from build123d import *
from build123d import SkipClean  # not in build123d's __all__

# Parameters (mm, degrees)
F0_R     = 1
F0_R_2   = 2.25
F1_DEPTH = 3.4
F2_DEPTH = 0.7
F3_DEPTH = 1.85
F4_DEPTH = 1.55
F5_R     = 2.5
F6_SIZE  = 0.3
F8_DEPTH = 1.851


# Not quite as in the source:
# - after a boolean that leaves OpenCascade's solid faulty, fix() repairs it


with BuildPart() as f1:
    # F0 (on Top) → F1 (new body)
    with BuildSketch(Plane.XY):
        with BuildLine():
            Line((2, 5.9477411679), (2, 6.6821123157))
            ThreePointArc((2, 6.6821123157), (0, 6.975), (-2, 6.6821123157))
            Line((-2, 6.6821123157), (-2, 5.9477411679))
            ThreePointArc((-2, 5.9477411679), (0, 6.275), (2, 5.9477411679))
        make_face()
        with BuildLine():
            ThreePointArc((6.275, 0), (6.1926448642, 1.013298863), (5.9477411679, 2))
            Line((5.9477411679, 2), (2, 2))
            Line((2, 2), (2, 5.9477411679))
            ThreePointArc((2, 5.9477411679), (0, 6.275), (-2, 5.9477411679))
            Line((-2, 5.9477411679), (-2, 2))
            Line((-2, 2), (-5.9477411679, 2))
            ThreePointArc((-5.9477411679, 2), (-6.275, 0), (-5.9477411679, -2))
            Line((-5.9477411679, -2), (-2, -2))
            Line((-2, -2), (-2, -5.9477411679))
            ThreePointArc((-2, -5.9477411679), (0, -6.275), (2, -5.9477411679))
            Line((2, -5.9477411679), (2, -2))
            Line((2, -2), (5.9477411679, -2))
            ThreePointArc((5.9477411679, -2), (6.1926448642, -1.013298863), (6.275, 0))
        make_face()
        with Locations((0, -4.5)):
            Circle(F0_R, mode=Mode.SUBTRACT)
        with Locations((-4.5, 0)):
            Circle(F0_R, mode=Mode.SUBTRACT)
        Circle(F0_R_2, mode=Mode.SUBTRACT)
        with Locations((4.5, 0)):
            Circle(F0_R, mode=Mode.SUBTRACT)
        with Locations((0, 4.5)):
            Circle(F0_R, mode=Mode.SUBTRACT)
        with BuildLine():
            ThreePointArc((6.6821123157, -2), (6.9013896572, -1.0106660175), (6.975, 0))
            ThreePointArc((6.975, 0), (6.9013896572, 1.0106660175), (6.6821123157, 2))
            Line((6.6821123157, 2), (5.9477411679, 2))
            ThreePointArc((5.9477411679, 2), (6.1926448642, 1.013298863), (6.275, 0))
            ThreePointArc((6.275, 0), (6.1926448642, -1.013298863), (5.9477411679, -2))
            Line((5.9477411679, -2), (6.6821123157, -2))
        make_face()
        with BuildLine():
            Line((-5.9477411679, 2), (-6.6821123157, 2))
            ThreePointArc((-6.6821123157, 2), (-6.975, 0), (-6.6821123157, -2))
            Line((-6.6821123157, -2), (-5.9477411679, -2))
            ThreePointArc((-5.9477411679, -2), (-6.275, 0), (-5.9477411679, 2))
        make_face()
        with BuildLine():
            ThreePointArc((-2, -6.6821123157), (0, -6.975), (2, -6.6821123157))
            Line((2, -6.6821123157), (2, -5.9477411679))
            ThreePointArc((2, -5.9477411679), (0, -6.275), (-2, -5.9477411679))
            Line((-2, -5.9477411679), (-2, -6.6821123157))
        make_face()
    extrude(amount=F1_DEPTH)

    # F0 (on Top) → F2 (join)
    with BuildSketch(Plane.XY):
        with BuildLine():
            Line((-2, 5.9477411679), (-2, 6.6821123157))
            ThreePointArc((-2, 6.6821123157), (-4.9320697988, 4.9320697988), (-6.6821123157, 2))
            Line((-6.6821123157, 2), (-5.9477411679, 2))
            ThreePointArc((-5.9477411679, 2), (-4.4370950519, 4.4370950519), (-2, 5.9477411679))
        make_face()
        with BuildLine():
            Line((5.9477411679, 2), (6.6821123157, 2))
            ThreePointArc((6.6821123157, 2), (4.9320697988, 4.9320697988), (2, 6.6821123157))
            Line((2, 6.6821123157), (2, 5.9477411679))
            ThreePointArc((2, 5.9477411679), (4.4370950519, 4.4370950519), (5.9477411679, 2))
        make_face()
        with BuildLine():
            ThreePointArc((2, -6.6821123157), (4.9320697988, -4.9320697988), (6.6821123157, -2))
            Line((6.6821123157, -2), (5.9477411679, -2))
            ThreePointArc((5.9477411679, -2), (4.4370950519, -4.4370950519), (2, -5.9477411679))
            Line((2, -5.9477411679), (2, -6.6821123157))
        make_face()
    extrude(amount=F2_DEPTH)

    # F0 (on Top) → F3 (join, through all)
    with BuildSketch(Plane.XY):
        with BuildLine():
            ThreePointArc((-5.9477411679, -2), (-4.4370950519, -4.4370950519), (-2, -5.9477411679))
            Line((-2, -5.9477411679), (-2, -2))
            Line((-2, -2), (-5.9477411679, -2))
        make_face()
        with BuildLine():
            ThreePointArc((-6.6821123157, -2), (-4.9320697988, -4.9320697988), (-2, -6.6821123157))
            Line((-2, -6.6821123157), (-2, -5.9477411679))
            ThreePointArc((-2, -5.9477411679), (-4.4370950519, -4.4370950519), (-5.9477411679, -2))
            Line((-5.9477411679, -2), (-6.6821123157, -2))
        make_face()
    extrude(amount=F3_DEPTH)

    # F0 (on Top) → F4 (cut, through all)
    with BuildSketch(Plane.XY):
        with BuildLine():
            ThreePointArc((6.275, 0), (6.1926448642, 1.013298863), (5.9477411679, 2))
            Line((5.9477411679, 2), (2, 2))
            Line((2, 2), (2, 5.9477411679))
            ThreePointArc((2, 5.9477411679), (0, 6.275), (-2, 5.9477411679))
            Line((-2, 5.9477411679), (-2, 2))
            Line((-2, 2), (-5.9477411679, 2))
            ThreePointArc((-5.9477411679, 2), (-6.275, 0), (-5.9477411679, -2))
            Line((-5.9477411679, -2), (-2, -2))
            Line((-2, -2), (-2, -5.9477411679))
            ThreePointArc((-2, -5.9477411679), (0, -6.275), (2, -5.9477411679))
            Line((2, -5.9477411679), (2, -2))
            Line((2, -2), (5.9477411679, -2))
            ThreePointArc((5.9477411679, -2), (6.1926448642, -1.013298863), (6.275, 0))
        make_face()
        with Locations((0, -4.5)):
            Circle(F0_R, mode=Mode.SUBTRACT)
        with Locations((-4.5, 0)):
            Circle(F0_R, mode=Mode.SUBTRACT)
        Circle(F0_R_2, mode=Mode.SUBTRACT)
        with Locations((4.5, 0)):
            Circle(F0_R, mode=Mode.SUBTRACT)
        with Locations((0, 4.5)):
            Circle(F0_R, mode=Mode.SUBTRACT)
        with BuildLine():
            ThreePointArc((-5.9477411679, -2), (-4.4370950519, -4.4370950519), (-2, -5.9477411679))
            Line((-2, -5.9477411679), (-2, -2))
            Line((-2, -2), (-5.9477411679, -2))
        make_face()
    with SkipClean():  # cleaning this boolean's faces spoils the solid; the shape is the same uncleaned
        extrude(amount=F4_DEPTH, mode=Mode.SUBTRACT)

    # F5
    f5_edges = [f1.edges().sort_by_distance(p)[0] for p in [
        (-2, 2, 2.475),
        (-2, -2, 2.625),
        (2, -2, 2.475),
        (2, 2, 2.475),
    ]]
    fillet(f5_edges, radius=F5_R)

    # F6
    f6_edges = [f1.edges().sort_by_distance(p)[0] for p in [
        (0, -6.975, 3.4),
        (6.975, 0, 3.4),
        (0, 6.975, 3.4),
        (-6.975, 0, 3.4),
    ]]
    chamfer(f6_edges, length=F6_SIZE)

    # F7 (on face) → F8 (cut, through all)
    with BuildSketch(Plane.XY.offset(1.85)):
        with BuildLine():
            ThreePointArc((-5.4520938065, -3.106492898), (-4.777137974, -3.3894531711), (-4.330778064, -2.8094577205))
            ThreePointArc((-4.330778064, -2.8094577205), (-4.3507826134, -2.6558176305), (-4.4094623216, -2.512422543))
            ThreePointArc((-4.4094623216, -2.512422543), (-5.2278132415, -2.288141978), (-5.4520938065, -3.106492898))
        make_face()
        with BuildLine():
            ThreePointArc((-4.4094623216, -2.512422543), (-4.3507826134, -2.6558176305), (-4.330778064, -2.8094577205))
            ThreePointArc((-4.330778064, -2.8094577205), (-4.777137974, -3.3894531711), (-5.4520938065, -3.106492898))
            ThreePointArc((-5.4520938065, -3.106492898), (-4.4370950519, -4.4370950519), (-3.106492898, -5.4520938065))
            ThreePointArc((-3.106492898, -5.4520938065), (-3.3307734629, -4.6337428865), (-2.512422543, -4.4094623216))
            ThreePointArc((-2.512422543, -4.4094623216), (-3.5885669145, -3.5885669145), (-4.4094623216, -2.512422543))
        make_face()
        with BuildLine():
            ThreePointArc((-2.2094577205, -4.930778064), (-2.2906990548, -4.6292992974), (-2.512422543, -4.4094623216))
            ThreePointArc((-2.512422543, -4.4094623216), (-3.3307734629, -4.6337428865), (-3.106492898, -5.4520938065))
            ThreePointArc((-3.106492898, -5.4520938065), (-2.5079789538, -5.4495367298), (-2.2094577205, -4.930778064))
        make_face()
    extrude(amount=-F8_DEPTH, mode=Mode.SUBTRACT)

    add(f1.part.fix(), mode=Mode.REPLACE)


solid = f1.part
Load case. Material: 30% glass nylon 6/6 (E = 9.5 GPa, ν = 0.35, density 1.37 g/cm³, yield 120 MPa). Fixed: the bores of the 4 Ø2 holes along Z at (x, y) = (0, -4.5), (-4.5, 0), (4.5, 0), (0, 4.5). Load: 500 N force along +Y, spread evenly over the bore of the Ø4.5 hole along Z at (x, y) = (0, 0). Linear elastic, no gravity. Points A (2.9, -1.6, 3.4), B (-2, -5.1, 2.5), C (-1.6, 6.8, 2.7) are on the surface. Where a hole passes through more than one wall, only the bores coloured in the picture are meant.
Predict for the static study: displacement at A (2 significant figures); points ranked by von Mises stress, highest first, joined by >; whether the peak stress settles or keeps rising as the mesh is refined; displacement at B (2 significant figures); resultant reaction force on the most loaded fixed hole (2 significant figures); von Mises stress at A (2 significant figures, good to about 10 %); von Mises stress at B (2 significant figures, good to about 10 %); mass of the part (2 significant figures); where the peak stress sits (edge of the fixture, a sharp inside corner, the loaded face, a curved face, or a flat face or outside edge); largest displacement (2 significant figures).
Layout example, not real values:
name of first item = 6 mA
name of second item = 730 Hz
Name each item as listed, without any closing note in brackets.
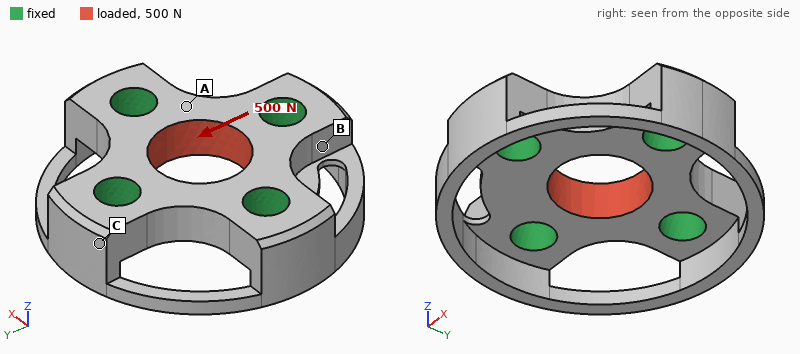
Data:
displacement at A = 5.6 µm
points ranked by von Mises stress, highest first, joined by > = A > B > C
whether the peak stress settles or keeps rising as the mesh is refined = keeps rising
displacement at B = 1.4 µm
resultant reaction force on the most loaded fixed hole = 170 N
von Mises stress at A = 14 MPa
von Mises stress at B = 8.8 MPa
mass of the part = 0.23 g
where the peak stress sits = edge of the fixture
largest displacement = 8.8 µm
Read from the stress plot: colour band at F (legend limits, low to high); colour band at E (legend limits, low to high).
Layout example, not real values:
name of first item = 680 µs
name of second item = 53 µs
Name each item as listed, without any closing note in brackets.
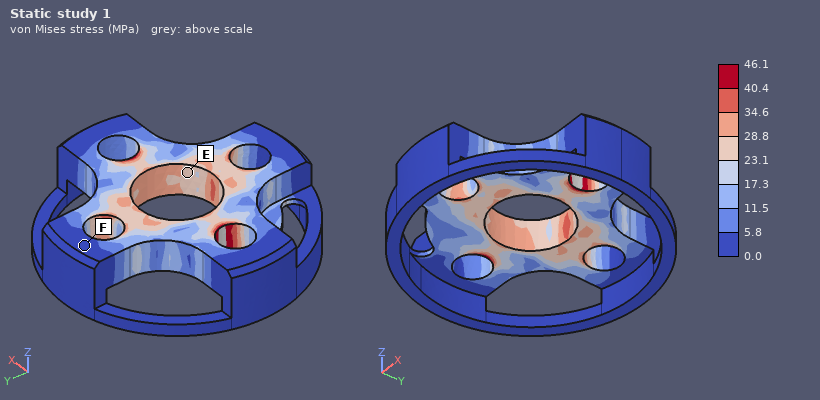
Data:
colour band at F = 0.0 to 5.8 MPa
colour band at E = 23.1 to 28.8 MPa
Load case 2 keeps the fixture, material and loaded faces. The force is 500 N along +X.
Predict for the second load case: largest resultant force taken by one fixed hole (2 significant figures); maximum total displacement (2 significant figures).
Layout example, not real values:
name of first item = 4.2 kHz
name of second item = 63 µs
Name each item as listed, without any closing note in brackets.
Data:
largest resultant force taken by one fixed hole = 170 N
maximum total displacement = 8.8 µm
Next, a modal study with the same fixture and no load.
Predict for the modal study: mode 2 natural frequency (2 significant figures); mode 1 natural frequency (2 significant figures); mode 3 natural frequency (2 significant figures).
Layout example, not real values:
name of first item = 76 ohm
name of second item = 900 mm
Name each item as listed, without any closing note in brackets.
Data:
mode 2 natural frequency = 32 kHz
mode 1 natural frequency = 31 kHz
mode 3 natural frequency = 32 kHz
